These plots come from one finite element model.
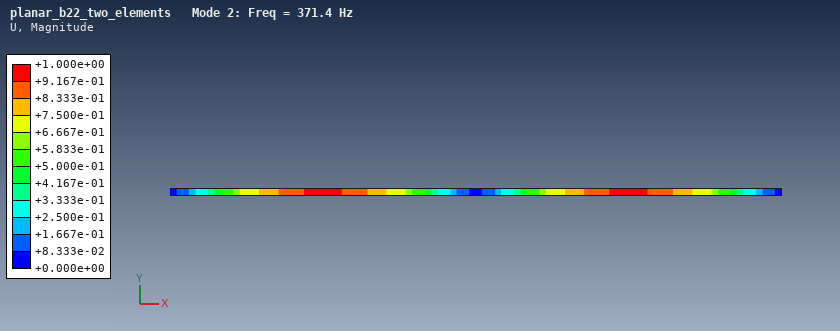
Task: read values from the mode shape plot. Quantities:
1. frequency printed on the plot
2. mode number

371.4 Hz
2
